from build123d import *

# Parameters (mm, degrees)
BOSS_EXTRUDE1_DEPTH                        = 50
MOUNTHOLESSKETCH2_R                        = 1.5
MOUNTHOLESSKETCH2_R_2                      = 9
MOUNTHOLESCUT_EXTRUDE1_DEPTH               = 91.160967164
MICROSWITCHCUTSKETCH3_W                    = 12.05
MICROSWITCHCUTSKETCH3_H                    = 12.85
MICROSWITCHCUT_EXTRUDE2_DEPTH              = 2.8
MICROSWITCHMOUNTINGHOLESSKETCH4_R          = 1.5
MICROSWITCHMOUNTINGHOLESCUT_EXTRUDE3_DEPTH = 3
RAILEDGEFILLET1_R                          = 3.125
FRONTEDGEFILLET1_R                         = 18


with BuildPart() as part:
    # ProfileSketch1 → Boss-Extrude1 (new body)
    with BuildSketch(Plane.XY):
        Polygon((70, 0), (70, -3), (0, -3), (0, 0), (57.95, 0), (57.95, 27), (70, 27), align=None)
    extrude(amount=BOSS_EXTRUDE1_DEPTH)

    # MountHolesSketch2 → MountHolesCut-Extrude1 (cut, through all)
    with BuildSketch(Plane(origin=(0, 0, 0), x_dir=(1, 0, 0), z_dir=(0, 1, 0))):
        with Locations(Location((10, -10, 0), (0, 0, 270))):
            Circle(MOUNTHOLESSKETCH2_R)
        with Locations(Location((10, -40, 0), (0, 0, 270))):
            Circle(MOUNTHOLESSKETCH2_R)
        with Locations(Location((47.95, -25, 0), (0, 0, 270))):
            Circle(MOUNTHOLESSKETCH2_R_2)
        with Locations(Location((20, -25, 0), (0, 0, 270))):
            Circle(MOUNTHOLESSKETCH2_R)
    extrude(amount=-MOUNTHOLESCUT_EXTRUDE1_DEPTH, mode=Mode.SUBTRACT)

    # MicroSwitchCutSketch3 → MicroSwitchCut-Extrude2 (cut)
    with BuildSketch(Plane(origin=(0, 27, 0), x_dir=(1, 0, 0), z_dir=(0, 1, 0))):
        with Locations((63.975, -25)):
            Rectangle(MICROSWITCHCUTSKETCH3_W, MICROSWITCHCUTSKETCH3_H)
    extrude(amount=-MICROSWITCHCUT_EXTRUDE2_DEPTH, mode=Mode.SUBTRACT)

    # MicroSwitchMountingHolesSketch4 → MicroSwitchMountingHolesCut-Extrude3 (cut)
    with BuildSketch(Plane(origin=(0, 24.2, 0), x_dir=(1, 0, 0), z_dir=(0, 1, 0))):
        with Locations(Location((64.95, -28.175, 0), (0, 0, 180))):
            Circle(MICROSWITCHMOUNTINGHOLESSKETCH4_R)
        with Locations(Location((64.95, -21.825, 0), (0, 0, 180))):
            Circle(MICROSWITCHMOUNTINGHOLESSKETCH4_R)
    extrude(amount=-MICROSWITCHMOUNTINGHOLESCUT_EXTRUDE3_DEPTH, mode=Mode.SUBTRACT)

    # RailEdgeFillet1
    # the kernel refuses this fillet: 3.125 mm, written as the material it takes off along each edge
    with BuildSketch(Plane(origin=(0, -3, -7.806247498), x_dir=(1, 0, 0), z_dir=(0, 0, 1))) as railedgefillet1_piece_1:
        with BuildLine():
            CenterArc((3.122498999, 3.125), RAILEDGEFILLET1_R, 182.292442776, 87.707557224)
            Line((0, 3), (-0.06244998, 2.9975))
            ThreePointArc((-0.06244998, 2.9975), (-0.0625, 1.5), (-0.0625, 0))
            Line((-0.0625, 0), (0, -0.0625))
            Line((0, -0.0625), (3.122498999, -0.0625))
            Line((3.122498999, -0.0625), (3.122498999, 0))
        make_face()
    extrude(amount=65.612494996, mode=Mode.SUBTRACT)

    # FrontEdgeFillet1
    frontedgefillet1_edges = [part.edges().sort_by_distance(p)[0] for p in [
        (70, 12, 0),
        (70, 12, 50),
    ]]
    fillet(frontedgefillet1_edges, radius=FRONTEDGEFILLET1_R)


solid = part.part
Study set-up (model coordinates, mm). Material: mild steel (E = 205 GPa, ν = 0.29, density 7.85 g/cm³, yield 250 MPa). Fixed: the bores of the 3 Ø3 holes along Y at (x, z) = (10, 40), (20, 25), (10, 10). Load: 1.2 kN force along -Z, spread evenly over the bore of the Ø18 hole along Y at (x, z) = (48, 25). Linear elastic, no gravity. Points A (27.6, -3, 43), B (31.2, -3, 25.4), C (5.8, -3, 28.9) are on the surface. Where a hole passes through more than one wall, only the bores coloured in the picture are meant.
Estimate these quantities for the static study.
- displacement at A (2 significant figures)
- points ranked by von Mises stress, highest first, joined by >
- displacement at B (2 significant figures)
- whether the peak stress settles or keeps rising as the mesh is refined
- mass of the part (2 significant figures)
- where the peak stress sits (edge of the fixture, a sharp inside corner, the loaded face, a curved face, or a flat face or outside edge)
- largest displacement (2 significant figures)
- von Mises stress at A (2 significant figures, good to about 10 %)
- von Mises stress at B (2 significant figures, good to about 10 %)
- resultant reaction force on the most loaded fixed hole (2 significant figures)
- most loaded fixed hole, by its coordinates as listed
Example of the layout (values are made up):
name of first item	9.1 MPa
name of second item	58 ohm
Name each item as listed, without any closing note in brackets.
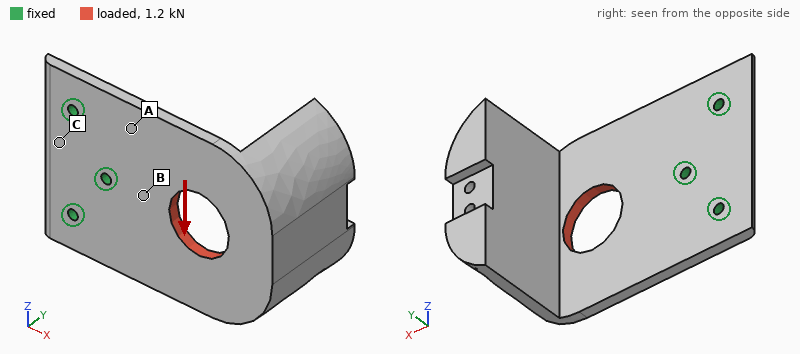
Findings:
displacement at A	3.6 µm
points ranked by von Mises stress, highest first, joined by >	B > A > C
displacement at B	3.5 µm
whether the peak stress settles or keeps rising as the mesh is refined	keeps rising
mass of the part	170 g
where the peak stress sits	edge of the fixture
largest displacement	15 µm
von Mises stress at A	16 MPa
von Mises stress at B	26 MPa
resultant reaction force on the most loaded fixed hole	1.2 kN
most loaded fixed hole, by its coordinates as listed	(20, 25)
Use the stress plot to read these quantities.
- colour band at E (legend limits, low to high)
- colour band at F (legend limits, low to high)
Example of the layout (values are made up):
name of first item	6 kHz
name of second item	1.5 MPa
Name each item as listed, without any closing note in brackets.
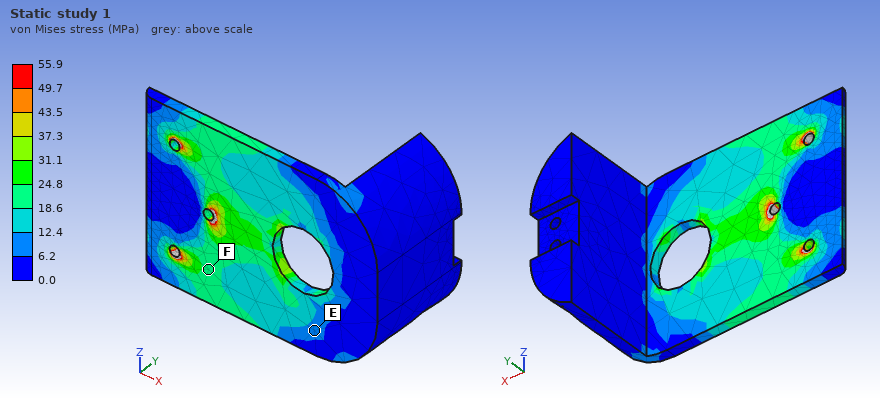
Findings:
colour band at E	6.2 to 12.4 MPa
colour band at F	18.6 to 24.8 MPa
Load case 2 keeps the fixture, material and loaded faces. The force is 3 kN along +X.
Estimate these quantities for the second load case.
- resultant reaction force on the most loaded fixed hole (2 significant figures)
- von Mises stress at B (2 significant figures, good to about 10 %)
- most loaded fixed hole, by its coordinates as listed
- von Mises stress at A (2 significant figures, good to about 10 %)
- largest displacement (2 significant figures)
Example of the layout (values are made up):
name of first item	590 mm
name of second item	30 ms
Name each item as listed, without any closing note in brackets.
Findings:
resultant reaction force on the most loaded fixed hole	1.2 kN
von Mises stress at B	26 MPa
most loaded fixed hole, by its coordinates as listed	(20, 25)
von Mises stress at A	18 MPa
largest displacement	6.6 µm
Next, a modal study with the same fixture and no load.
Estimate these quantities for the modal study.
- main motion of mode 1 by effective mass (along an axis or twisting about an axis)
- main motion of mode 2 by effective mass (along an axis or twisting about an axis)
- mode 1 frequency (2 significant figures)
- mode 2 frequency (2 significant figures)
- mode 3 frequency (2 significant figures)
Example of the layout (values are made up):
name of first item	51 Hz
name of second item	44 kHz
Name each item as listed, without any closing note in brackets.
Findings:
main motion of mode 1 by effective mass	along Y
main motion of mode 2 by effective mass	along Z
mode 1 frequency	340 Hz
mode 2 frequency	790 Hz
mode 3 frequency	1500 Hz
